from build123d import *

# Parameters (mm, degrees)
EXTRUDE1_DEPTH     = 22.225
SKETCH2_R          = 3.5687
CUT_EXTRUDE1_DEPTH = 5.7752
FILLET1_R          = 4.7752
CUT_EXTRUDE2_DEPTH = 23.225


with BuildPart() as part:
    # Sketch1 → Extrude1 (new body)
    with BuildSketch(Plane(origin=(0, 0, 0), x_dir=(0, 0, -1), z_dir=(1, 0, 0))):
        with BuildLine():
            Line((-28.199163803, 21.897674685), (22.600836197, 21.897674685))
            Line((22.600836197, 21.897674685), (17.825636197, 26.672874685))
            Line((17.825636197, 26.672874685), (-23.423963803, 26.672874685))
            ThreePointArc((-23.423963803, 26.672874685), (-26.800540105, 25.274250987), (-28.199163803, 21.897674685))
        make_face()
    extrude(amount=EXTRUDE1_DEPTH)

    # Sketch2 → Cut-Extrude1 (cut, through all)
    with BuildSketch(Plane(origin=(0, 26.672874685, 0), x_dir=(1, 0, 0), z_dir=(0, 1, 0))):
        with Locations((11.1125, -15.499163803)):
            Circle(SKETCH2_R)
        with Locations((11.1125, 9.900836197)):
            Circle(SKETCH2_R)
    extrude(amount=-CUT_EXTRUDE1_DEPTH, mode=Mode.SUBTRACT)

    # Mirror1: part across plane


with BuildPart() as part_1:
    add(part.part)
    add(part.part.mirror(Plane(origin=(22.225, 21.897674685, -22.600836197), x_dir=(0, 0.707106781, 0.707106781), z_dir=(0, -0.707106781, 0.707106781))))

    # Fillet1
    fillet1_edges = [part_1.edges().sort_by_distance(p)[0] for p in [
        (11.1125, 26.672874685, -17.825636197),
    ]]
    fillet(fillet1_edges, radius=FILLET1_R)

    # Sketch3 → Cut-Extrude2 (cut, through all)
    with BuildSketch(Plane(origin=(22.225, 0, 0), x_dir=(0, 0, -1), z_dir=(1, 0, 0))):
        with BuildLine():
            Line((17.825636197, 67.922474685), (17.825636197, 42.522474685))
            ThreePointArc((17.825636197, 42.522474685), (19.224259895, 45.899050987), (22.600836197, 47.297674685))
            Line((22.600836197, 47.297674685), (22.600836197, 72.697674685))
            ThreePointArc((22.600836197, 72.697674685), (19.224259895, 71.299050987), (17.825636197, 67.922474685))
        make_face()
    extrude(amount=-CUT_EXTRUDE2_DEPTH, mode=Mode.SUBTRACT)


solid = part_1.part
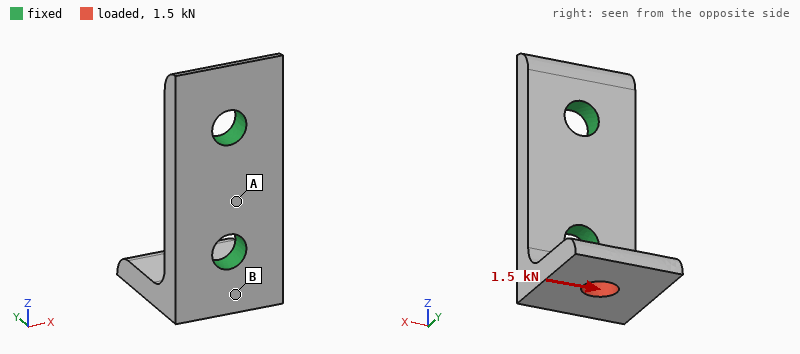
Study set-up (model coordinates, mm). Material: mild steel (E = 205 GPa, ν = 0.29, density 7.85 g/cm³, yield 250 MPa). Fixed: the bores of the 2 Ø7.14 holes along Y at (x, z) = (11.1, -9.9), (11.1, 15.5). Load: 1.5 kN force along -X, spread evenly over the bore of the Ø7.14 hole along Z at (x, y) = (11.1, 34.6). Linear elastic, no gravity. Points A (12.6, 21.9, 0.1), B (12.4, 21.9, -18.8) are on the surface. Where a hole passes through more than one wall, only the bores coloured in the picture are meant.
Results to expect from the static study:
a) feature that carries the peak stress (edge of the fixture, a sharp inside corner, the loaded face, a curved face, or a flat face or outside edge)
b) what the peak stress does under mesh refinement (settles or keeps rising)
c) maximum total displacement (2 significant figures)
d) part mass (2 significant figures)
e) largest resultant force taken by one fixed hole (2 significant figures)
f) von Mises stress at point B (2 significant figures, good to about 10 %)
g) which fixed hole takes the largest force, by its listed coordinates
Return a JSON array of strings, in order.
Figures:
["edge of the fixture", "keeps rising", "33 µm", "54 g", "1.7 kN", "44 MPa", "(11.1, -9.9)"]
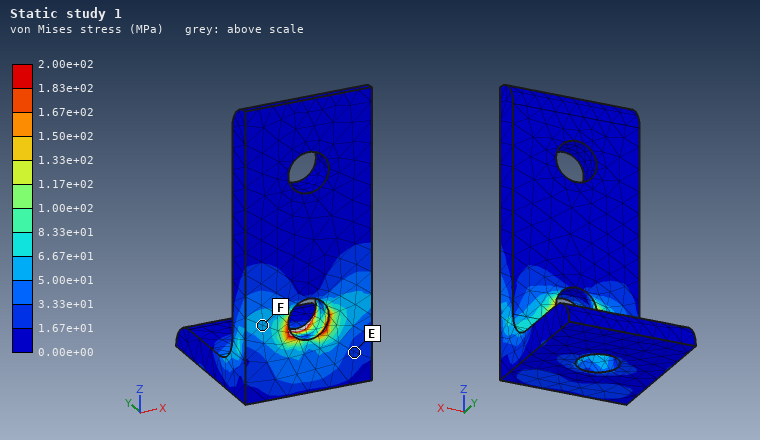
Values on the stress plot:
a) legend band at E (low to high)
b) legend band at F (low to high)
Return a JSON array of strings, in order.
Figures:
["1.67e+01 to 3.33e+01 MPa", "5.00e+01 to 6.67e+01 MPa"]
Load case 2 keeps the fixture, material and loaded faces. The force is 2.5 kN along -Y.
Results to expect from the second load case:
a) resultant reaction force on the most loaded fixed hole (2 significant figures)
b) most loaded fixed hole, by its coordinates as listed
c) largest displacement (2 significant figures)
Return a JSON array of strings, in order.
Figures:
["2.6 kN", "(11.1, -9.9)", "51 µm"]
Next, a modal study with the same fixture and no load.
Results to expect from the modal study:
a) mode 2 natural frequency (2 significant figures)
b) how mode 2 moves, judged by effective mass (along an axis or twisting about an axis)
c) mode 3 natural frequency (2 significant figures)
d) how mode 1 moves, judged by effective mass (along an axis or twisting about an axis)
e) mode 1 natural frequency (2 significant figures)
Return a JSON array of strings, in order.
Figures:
["8800 Hz", "along X", "16 kHz", "along Z", "6100 Hz"]
